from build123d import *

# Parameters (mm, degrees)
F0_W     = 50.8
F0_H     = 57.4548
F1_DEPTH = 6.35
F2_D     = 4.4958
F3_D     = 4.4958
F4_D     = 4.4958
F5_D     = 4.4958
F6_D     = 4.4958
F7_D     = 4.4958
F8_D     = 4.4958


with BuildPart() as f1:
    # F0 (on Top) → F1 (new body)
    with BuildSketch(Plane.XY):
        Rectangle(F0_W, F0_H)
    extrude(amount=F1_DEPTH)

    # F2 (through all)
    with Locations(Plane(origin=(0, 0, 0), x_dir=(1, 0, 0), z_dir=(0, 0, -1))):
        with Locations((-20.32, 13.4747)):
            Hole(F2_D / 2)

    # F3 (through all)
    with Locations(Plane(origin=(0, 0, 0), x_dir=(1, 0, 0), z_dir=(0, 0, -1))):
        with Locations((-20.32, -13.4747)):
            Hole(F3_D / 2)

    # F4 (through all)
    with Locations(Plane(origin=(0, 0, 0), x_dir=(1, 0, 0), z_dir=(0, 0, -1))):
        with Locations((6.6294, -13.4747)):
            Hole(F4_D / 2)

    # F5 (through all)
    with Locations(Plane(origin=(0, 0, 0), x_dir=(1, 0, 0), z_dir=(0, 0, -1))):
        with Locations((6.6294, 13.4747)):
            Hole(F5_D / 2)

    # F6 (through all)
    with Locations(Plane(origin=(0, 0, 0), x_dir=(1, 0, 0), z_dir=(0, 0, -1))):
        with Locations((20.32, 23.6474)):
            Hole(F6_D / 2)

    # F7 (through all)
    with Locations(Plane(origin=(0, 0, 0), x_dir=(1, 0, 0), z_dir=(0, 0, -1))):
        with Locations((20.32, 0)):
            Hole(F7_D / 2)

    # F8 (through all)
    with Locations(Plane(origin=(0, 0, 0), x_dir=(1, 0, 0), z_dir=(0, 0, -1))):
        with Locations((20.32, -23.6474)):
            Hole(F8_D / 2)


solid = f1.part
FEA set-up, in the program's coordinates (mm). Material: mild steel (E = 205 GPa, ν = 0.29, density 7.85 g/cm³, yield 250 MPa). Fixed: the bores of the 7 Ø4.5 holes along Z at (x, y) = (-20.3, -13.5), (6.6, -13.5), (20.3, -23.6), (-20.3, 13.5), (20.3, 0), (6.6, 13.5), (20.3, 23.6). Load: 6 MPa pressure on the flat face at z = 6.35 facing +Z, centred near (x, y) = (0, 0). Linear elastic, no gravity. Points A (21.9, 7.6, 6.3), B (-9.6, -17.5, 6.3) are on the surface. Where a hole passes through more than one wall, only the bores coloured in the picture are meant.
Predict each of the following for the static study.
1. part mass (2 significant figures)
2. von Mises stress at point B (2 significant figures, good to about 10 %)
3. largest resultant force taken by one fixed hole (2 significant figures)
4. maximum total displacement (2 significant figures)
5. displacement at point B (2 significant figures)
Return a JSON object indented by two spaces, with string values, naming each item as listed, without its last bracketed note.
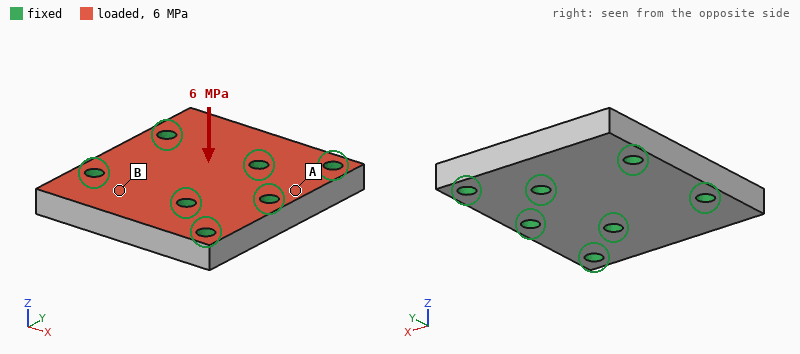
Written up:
{
  "part mass": "140 g",
  "von Mises stress at point B": "44 MPa",
  "largest resultant force taken by one fixed hole": "3.2 kN",
  "maximum total displacement": "12 µm",
  "displacement at point B": "5.4 µm"
}
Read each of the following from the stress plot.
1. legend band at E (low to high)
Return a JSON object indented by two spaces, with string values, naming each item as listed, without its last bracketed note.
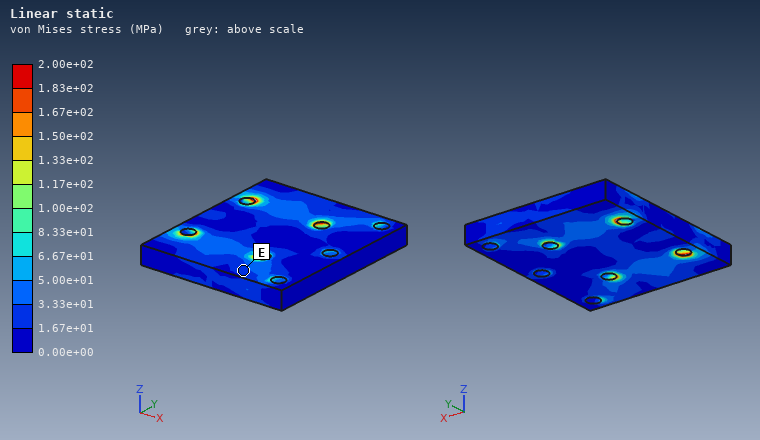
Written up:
{
  "legend band at E": "1.67e+01 to 3.33e+01 MPa"
}
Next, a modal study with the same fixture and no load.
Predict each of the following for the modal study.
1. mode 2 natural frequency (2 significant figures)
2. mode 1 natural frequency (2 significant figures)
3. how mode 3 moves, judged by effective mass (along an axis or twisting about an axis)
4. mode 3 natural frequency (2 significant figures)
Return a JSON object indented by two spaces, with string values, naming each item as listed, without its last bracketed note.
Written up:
{
  "mode 2 natural frequency": "20 kHz",
  "mode 1 natural frequency": "20 kHz",
  "how mode 3 moves, judged by effective mass": "along Z",
  "mode 3 natural frequency": "29 kHz"
}
